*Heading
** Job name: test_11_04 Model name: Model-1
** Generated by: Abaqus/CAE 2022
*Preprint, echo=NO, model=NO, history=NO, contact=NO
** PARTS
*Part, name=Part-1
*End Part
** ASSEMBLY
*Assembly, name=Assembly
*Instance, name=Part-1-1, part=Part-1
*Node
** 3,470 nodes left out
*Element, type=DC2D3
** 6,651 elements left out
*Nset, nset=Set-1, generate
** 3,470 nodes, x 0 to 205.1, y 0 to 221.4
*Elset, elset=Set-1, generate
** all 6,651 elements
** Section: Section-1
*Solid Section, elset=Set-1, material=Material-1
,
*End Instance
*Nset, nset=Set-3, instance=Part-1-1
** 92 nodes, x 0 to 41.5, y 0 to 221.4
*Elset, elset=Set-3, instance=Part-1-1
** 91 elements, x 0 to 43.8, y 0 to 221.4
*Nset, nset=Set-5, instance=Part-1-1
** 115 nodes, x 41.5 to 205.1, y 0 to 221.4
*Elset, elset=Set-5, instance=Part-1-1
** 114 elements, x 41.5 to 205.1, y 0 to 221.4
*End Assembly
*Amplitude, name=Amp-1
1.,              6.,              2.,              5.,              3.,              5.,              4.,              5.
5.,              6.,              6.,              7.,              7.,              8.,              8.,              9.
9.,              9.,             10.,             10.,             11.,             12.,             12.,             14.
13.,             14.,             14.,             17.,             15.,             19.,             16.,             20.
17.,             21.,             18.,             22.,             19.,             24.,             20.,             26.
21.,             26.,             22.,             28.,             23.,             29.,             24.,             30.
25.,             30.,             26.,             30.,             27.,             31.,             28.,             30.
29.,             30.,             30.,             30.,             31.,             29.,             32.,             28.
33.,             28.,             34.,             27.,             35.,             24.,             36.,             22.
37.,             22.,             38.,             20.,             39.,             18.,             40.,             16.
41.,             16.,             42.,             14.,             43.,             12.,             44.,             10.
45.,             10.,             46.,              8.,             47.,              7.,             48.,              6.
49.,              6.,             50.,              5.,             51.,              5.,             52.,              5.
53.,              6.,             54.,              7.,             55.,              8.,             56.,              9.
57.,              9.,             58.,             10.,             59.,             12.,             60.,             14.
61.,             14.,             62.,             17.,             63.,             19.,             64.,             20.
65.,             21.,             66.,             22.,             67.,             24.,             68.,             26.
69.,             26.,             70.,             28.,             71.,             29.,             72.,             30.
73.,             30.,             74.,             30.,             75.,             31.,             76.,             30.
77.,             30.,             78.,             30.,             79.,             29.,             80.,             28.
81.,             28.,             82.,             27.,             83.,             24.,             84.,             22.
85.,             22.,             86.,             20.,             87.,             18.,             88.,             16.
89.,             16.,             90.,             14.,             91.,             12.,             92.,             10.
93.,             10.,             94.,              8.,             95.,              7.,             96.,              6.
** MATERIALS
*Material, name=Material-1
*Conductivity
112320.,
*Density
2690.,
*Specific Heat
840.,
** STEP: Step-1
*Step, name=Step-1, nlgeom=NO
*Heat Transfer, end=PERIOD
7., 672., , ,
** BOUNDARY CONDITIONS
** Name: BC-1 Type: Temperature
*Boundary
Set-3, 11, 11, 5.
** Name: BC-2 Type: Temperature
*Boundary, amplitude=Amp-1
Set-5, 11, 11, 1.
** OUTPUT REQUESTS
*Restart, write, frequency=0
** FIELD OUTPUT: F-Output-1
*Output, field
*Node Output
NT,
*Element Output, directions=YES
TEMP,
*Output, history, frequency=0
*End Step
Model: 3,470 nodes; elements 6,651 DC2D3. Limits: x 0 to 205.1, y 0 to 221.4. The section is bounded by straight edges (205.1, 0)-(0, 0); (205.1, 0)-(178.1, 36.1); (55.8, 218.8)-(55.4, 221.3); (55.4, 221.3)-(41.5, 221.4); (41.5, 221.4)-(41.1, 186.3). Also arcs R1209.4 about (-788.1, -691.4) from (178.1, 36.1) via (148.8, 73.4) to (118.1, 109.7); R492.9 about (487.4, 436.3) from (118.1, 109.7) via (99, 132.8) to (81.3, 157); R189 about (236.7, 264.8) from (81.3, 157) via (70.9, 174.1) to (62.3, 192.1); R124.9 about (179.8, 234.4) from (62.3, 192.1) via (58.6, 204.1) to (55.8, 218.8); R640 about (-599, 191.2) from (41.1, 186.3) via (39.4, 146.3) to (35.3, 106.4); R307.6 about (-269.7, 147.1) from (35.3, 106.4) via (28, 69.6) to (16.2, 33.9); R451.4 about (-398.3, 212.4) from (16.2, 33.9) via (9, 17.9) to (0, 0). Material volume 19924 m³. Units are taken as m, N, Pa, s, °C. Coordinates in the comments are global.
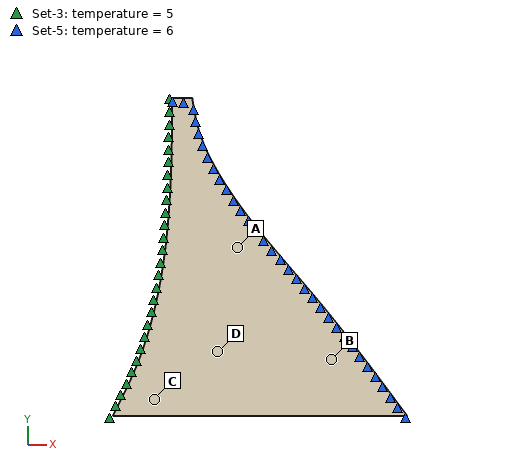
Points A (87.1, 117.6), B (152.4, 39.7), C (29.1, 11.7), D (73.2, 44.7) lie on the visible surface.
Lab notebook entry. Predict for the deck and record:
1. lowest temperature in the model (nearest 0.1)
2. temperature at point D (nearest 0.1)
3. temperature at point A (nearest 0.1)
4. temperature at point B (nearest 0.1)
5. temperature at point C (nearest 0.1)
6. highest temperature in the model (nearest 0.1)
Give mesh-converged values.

0.0 °C
0.0 °C
0.2 °C
0.3 °C
0.1 °C
6.0 °C
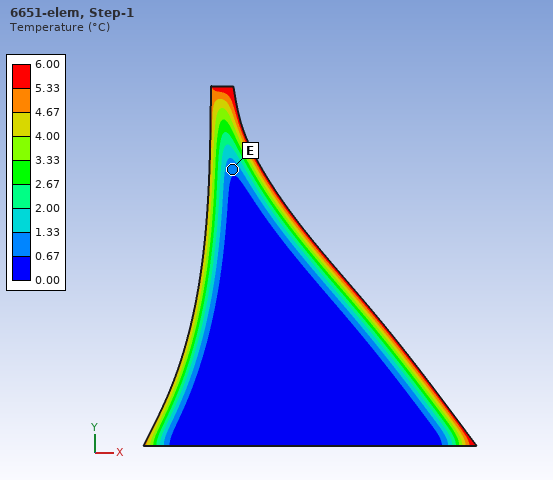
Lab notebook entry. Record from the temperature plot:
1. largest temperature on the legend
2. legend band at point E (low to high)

6.00 °C
0.67 to 1.33 °C
